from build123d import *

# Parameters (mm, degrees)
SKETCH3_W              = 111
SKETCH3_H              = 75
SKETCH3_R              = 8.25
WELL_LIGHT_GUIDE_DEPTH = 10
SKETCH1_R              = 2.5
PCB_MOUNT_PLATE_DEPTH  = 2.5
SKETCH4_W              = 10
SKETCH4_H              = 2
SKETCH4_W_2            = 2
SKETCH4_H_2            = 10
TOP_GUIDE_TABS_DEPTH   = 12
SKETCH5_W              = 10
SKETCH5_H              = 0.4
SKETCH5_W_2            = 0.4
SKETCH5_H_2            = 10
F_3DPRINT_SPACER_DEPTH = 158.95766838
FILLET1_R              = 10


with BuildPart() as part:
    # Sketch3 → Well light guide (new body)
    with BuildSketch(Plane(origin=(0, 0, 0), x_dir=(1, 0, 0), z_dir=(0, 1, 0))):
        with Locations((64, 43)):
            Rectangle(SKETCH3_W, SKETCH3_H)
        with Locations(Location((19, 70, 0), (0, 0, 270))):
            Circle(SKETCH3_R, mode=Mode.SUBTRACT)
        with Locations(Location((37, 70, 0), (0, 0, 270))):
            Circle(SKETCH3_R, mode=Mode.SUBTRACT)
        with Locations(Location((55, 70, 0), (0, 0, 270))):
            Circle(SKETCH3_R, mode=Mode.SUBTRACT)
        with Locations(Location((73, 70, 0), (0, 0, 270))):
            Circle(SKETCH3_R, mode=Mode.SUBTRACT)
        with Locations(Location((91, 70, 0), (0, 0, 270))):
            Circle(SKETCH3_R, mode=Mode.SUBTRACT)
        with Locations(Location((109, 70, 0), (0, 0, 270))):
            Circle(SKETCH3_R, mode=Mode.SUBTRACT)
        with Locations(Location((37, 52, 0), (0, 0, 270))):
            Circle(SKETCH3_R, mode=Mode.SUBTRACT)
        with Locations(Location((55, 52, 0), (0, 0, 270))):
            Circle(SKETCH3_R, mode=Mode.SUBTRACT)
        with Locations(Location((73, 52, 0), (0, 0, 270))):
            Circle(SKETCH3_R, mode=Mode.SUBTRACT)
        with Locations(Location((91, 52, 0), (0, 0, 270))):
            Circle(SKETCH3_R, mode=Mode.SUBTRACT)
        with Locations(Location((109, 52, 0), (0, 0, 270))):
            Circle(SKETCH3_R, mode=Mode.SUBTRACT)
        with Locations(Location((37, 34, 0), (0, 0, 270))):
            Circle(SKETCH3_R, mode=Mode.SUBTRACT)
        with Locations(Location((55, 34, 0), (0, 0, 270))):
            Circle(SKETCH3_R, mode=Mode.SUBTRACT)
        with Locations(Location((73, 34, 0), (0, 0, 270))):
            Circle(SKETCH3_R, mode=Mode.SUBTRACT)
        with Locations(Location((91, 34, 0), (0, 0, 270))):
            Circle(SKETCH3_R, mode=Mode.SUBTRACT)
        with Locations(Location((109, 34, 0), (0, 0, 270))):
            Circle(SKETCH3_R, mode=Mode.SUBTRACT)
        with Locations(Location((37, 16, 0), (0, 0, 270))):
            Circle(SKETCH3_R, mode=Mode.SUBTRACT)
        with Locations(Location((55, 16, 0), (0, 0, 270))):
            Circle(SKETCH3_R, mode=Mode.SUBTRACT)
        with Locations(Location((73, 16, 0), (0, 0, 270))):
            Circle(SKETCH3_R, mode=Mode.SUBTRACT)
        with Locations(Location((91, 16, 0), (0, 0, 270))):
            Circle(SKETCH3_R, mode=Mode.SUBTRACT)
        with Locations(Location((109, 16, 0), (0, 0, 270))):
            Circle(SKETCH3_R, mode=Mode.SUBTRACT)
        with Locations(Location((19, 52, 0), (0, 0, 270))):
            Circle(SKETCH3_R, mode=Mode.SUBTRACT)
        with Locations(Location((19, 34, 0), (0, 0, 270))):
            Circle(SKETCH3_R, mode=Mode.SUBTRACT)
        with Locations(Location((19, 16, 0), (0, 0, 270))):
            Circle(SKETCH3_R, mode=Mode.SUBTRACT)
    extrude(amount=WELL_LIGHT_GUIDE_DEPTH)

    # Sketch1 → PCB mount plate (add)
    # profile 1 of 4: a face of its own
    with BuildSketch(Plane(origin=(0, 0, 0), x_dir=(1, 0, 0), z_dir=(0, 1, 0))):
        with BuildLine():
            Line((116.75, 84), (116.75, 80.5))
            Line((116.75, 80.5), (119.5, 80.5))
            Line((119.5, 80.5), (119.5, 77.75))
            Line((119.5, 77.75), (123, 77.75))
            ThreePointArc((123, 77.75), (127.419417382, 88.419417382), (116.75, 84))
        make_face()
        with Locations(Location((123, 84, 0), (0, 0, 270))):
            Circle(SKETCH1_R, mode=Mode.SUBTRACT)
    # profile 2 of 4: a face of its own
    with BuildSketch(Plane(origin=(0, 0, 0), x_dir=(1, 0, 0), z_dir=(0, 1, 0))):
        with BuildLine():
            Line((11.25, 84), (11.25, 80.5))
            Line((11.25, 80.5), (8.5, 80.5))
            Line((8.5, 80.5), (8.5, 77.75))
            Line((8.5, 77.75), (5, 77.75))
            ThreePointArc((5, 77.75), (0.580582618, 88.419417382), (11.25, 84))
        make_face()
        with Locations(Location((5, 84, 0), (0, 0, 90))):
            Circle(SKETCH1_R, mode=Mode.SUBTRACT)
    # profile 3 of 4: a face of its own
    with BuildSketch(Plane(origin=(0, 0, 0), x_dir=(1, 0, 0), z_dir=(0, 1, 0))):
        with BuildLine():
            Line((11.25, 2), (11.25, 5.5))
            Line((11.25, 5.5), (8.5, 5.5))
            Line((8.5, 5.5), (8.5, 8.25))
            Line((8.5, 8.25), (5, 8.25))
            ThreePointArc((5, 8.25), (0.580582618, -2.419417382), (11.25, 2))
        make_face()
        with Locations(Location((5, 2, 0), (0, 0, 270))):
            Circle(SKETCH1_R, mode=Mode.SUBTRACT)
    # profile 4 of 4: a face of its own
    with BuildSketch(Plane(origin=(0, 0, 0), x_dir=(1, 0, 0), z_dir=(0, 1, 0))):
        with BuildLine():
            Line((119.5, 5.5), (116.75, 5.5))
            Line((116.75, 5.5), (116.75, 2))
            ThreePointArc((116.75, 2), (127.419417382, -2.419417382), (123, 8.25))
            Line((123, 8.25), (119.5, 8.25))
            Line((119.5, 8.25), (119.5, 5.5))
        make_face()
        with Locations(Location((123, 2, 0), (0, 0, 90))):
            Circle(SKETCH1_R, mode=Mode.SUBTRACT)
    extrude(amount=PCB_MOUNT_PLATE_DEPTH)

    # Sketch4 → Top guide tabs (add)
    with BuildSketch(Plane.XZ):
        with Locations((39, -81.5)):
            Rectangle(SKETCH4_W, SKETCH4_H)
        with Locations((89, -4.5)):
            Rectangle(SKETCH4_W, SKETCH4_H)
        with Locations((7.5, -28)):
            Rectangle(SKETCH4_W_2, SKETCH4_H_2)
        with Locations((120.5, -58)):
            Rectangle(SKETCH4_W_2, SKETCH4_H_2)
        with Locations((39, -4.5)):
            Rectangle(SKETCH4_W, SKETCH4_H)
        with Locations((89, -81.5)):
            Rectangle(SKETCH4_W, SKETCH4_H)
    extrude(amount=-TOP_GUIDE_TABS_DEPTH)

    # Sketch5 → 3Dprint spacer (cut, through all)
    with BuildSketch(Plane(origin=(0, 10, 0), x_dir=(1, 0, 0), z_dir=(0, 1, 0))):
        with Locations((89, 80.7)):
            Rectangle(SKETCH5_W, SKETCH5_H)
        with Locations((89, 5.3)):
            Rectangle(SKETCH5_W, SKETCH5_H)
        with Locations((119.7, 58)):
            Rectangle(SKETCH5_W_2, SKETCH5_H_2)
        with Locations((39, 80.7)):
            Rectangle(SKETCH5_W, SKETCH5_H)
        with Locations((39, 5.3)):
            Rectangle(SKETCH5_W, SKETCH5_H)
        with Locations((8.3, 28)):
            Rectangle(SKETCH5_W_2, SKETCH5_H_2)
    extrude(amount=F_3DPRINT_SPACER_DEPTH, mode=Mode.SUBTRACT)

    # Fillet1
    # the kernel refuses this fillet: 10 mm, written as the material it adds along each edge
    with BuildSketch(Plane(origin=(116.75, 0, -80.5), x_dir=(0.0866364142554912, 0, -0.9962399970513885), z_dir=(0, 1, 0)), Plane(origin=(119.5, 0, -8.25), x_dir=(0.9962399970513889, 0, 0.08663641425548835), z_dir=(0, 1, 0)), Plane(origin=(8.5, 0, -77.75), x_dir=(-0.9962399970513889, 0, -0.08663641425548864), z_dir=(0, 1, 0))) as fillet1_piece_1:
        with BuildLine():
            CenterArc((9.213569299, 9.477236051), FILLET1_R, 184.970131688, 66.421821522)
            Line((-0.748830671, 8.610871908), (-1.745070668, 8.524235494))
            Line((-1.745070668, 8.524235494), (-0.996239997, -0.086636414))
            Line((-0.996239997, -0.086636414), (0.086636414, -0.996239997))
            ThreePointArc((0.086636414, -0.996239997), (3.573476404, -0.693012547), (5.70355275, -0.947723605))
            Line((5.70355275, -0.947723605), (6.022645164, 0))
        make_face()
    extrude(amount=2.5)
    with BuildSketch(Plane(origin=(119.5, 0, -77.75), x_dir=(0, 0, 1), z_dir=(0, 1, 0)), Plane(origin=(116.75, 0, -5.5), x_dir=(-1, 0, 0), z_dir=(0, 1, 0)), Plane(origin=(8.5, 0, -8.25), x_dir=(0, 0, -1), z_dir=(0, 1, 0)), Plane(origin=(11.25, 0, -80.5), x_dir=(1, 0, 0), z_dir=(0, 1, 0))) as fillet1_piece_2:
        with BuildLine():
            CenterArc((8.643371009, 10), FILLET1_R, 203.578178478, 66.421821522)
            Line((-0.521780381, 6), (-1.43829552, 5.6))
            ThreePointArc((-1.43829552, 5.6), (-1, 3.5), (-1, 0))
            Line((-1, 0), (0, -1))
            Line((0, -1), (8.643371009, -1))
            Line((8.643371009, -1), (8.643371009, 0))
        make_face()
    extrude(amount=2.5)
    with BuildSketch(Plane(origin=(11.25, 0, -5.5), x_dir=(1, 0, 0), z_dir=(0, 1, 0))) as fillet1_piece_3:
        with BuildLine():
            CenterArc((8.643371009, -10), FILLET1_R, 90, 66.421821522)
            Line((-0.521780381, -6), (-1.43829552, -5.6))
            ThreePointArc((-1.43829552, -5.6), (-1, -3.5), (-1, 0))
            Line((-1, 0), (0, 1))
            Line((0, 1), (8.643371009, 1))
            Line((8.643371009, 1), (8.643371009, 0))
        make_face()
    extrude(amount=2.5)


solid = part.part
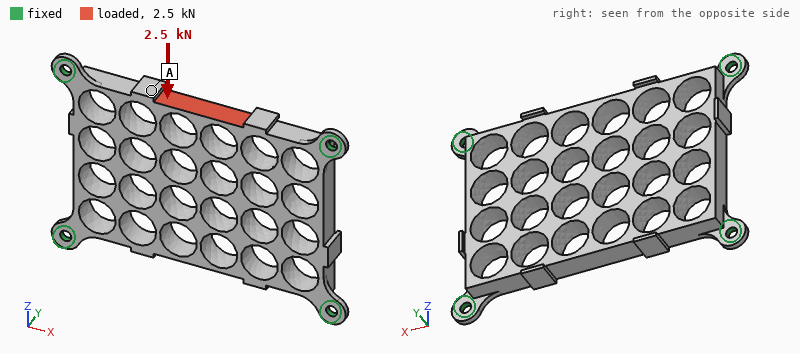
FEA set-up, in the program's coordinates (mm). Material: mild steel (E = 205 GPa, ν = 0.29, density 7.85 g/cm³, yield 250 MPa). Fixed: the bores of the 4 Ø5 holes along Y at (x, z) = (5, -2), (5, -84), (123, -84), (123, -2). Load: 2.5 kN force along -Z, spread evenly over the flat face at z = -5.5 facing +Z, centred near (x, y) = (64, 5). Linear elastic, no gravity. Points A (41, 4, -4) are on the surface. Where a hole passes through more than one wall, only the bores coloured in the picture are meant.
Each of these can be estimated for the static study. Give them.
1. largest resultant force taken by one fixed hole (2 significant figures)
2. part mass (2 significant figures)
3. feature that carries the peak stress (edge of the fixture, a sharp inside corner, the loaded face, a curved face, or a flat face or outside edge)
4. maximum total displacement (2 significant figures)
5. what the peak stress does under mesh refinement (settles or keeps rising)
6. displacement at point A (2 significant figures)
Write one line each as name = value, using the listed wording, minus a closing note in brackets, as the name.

largest resultant force taken by one fixed hole = 740 N
part mass = 270 g
feature that carries the peak stress = a sharp inside corner
maximum total displacement = 47 µm
what the peak stress does under mesh refinement = keeps rising
displacement at point A = 32 µm
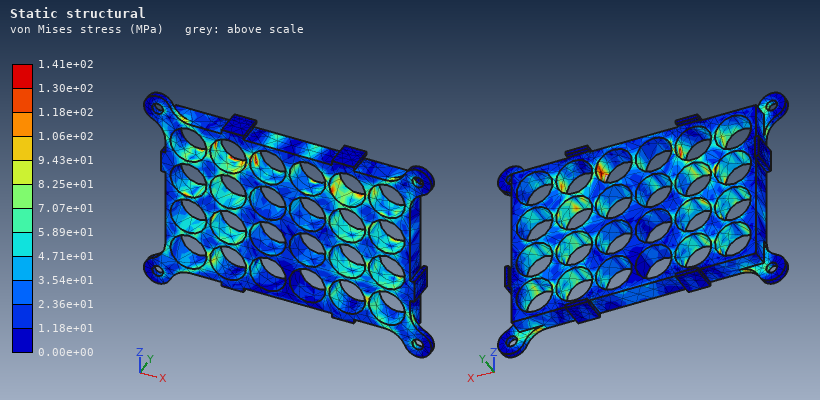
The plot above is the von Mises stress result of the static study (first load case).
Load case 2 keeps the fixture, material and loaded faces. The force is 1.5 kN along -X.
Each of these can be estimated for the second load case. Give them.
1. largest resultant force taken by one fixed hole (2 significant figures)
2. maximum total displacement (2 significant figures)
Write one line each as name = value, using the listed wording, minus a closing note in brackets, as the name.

largest resultant force taken by one fixed hole = 670 N
maximum total displacement = 9.7 µm
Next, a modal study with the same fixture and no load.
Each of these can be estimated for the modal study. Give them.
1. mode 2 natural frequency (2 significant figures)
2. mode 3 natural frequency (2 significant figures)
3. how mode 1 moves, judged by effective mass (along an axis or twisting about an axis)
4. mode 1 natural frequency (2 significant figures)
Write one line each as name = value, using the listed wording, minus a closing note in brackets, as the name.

mode 2 natural frequency = 2300 Hz
mode 3 natural frequency = 3400 Hz
how mode 1 moves, judged by effective mass = along Y
mode 1 natural frequency = 1600 Hz
